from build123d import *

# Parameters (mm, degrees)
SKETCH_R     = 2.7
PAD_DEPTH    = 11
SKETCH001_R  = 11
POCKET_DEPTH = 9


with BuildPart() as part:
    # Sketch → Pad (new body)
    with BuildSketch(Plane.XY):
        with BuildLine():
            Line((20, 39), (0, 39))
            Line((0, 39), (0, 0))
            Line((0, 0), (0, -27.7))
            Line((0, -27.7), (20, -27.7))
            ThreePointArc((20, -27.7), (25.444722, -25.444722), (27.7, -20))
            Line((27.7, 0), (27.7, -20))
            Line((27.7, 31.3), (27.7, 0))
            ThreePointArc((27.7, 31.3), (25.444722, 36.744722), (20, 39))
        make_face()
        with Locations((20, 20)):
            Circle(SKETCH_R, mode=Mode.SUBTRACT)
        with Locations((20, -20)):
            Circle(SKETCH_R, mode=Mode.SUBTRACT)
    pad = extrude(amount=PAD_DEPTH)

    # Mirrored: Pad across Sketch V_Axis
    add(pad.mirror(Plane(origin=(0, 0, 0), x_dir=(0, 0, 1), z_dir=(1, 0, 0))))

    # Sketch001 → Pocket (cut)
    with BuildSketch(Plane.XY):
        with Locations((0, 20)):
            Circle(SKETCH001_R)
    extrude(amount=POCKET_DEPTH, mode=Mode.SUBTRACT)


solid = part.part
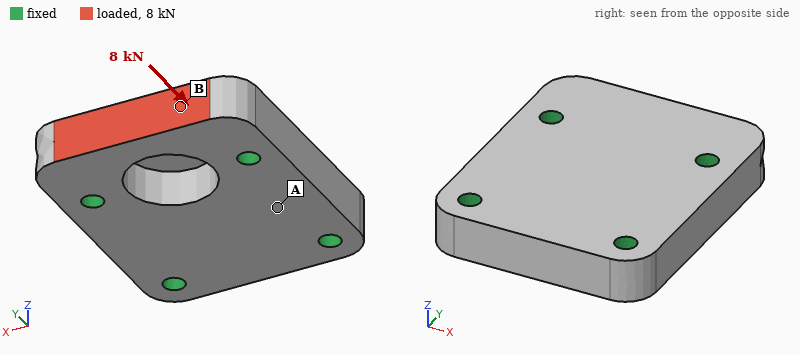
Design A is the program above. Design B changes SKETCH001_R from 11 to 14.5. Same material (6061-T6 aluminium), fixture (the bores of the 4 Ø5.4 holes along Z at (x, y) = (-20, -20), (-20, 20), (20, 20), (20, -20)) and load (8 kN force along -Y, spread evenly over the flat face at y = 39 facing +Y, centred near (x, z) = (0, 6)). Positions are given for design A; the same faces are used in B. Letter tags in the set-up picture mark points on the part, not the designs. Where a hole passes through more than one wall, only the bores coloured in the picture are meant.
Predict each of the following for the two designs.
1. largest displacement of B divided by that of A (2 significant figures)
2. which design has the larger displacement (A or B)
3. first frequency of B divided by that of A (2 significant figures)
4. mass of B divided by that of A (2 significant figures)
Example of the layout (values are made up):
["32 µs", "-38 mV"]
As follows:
["2.0", "B", "0.96", "0.93"]
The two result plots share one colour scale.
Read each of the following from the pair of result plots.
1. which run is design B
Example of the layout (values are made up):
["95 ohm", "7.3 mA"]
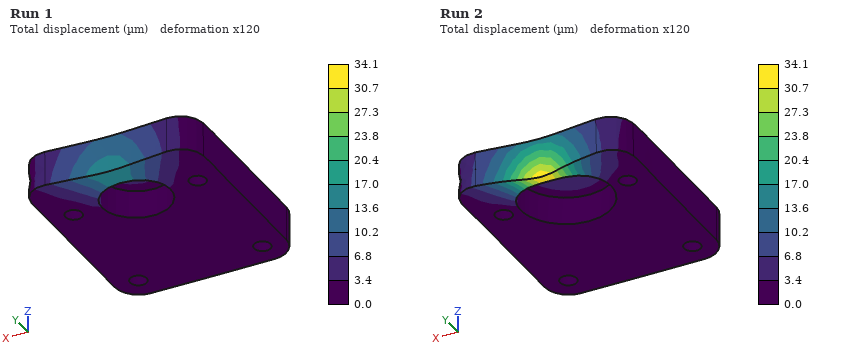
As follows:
["Run 2"]
